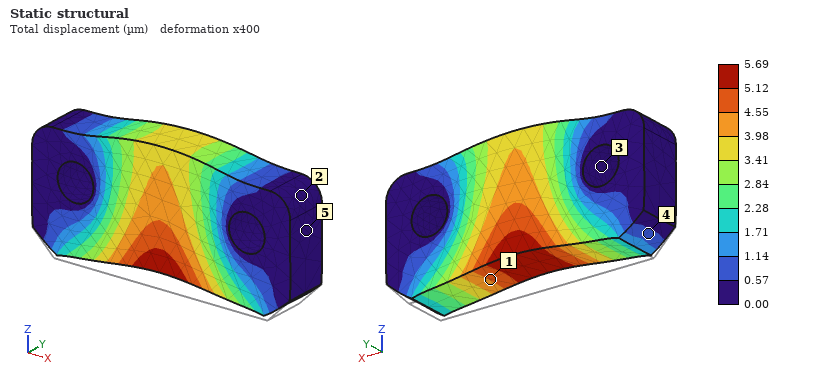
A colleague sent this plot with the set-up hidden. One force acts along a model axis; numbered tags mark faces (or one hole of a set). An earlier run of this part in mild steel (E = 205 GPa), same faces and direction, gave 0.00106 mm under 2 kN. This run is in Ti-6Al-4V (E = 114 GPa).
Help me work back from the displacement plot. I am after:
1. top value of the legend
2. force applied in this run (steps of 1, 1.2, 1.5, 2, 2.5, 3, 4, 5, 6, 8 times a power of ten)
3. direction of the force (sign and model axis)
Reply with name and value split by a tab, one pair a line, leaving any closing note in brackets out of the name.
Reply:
top value of the legend	5.69 µm
force applied in this run	6 kN
direction of the force	+Z
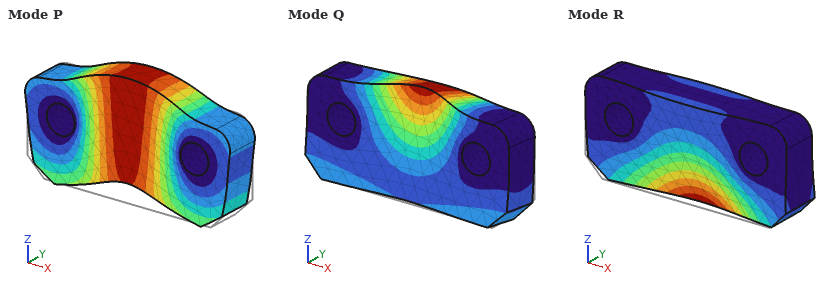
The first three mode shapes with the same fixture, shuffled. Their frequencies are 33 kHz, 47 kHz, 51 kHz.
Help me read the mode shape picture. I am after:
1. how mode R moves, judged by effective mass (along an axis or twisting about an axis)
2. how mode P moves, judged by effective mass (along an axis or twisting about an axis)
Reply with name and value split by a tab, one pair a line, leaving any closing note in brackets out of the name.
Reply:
how mode R moves, judged by effective mass	along Y
how mode P moves, judged by effective mass	along Z
